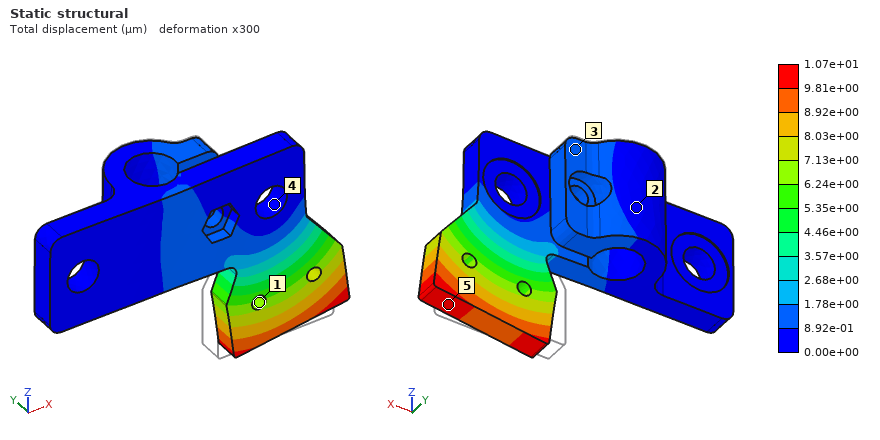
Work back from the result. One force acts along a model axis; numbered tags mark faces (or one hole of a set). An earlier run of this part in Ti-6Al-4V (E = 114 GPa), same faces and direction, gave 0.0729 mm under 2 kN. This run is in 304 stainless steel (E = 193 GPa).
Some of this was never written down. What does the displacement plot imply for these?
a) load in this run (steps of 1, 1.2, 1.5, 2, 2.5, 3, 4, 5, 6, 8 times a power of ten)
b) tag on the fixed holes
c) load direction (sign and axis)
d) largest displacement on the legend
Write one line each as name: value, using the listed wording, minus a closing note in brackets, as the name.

load in this run: 500 N
tag on the fixed holes: 4
load direction: +X
largest displacement on the legend: 1.07e+01 µm
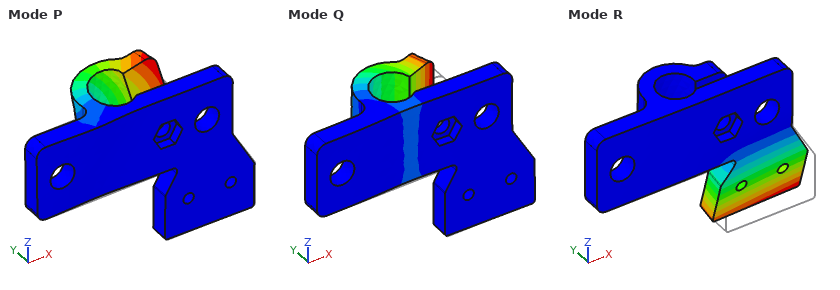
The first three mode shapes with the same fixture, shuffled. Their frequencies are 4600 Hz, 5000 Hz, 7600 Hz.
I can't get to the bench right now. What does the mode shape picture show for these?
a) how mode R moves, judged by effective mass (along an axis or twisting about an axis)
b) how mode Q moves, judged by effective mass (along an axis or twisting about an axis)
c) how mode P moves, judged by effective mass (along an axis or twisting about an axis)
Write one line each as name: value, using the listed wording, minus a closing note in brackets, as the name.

how mode R moves, judged by effective mass: along Y
how mode Q moves, judged by effective mass: along Y
how mode P moves, judged by effective mass: along Z
